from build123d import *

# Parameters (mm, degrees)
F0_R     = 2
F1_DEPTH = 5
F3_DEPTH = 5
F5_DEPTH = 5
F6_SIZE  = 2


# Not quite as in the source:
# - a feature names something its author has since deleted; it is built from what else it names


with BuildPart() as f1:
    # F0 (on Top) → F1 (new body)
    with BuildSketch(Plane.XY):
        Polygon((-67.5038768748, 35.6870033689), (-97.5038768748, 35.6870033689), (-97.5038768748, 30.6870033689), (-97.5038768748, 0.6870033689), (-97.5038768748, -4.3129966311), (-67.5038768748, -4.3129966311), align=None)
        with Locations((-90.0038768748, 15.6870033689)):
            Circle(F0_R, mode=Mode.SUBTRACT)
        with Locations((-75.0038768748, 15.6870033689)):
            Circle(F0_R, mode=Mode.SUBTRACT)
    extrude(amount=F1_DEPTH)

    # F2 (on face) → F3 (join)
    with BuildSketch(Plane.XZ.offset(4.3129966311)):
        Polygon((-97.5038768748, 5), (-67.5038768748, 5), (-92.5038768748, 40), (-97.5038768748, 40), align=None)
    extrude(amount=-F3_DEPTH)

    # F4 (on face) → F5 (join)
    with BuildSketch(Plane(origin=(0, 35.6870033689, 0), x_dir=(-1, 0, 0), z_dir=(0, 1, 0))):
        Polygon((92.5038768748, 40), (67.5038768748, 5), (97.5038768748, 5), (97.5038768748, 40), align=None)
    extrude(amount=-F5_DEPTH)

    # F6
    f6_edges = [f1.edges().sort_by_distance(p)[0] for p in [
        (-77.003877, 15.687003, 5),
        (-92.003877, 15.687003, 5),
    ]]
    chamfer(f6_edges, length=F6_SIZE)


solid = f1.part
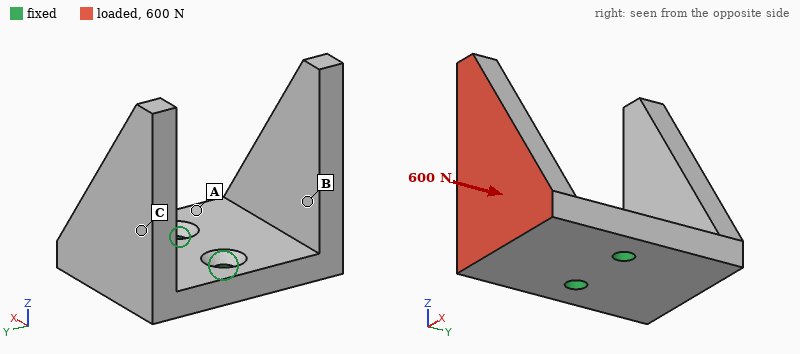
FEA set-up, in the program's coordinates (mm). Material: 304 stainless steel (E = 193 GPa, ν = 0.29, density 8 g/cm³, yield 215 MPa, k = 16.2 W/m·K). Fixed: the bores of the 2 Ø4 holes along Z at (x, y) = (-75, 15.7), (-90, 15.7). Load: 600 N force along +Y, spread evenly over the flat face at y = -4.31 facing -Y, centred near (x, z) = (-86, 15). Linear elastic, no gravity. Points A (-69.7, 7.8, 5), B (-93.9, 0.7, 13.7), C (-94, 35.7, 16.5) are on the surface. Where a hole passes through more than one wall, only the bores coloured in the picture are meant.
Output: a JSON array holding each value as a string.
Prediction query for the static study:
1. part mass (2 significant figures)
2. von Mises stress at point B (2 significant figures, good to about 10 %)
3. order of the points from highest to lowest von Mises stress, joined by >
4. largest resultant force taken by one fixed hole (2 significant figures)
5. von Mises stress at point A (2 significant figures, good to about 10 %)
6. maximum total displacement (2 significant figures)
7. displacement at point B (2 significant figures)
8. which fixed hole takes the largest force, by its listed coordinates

["95 g", "33 MPa", "A > B > C", "430 N", "58 MPa", "0.15 mm", "0.041 mm", "(-90, 15.7)"]
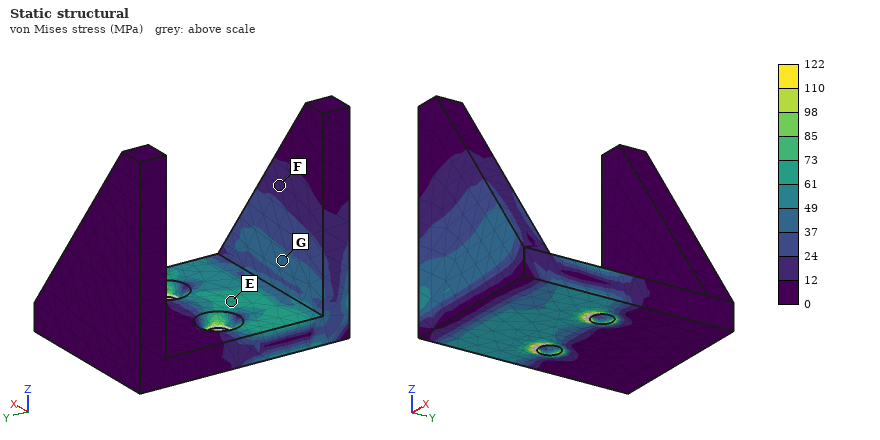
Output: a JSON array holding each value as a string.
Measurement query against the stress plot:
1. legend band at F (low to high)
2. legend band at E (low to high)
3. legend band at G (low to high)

["12 to 24 MPa", "61 to 73 MPa", "37 to 49 MPa"]
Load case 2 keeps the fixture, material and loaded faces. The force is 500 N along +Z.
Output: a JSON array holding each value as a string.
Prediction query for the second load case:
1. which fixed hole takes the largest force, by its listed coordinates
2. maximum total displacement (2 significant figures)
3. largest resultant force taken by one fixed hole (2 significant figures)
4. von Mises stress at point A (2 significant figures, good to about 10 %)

["(-90, 15.7)", "97 µm", "350 N", "48 MPa"]
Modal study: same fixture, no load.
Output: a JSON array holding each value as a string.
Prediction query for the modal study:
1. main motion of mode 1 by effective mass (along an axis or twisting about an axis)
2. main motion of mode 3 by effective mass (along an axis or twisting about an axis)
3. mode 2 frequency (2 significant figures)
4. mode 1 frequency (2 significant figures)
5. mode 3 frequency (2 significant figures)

["along Y", "twisting about Z", "2400 Hz", "2100 Hz", "4200 Hz"]
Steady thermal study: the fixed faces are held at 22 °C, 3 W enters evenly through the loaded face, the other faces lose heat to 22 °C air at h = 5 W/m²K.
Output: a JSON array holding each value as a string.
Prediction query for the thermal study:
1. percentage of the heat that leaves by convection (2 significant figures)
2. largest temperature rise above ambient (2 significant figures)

["8.6 %", "41 K"]
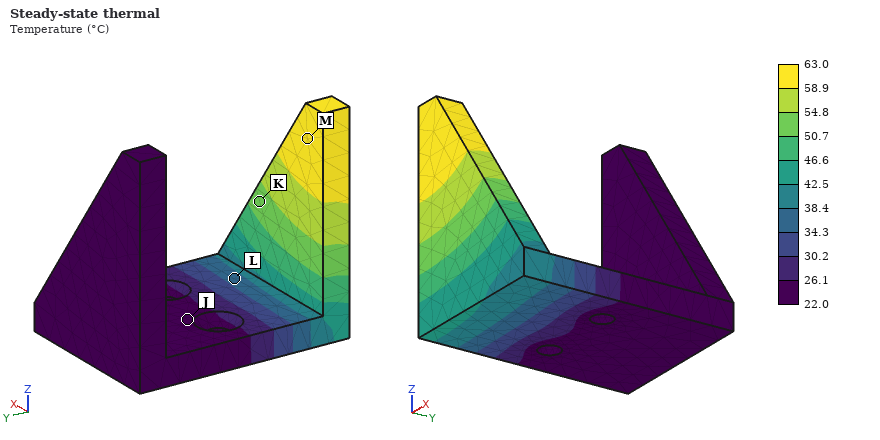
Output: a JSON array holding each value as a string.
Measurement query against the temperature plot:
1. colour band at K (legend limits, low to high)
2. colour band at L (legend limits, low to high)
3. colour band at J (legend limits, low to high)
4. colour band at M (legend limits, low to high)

["50.7 to 54.8 °C", "34.3 to 38.4 °C", "22.0 to 26.1 °C", "58.9 to 63.0 °C"]
